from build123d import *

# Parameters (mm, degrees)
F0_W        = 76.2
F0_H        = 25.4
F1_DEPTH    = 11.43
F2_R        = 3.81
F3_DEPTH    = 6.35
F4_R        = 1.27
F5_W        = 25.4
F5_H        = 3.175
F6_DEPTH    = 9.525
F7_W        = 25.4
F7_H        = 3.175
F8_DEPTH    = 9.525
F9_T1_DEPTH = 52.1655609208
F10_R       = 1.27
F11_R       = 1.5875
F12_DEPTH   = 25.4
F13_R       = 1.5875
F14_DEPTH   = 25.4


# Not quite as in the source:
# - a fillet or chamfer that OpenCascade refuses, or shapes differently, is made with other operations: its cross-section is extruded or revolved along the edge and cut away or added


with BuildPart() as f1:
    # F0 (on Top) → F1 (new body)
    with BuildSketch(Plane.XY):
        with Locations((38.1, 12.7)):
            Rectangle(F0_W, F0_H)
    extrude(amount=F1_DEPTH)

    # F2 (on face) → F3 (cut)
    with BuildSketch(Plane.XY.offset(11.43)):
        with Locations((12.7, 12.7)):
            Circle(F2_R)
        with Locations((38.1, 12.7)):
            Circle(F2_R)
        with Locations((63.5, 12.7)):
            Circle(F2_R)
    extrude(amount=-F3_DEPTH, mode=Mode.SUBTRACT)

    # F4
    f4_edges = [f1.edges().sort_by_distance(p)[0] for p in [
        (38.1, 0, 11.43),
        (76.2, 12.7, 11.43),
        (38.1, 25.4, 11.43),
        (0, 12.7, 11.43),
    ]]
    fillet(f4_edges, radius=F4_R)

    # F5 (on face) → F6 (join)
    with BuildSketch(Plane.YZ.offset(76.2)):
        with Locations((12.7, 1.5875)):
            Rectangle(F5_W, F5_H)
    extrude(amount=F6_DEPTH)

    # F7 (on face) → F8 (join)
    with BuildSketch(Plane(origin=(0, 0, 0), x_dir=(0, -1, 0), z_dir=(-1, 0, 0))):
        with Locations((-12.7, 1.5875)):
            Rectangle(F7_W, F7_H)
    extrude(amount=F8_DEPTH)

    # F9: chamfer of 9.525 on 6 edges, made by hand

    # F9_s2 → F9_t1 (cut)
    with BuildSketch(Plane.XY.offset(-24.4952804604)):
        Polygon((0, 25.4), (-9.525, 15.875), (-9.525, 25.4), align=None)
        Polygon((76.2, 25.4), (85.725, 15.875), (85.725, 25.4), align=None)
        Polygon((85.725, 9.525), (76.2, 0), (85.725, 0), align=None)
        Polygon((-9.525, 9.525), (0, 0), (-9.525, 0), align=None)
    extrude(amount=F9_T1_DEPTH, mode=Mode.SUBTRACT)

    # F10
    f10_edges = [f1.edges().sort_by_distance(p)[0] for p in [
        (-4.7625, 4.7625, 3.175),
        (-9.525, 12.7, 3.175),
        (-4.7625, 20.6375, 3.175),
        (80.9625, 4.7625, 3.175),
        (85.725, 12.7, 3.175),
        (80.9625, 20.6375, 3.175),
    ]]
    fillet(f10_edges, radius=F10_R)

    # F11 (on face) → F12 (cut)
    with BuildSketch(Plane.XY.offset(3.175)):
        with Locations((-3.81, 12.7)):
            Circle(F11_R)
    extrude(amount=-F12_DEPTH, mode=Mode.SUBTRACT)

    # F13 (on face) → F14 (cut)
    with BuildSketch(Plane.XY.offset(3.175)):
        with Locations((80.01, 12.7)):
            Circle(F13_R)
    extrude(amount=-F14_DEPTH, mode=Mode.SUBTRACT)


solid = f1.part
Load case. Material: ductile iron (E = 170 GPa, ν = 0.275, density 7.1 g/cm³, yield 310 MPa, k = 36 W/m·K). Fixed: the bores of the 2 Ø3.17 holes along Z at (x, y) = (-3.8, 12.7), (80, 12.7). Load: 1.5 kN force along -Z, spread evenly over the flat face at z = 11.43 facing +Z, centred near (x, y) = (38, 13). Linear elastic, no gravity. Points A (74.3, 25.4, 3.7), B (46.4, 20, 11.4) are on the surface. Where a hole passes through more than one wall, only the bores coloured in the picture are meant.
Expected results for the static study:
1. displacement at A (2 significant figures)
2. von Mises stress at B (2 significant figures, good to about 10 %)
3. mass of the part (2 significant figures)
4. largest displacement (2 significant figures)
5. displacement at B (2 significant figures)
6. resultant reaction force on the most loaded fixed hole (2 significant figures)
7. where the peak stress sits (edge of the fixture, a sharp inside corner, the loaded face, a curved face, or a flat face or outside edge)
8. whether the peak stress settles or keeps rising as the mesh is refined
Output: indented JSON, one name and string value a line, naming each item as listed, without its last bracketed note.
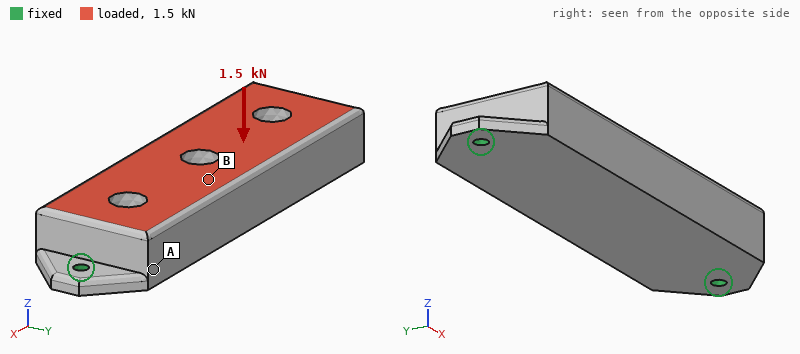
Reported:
{
  "displacement at A": "4.8 µm",
  "von Mises stress at B": "24 MPa",
  "mass of the part": "160 g",
  "largest displacement": "18 µm",
  "displacement at B": "16 µm",
  "resultant reaction force on the most loaded fixed hole": "1.3 kN",
  "where the peak stress sits": "edge of the fixture",
  "whether the peak stress settles or keeps rising as the mesh is refined": "keeps rising"
}
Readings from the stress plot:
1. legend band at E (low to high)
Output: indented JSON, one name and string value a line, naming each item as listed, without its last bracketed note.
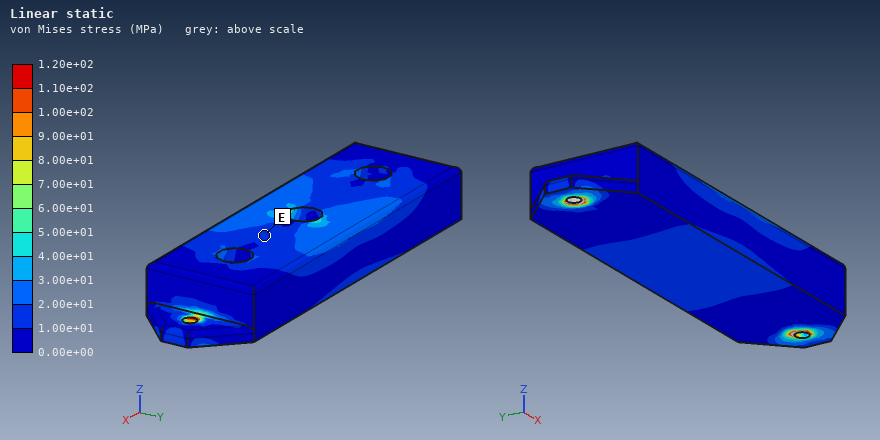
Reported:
{
  "legend band at E": "1.00e+01 to 2.00e+01 MPa"
}
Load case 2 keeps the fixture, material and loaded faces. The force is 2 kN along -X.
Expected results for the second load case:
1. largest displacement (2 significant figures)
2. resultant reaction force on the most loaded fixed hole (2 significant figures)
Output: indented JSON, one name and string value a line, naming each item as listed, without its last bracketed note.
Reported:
{
  "largest displacement": "2.1 µm",
  "resultant reaction force on the most loaded fixed hole": "1.0 kN"
}
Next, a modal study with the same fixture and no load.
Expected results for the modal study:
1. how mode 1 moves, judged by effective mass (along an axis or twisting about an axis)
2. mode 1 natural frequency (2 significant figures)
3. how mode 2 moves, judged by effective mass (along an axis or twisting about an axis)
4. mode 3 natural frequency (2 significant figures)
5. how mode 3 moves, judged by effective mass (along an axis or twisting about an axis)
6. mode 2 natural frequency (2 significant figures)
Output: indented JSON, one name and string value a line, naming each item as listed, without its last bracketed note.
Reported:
{
  "how mode 1 moves, judged by effective mass": "along Y",
  "mode 1 natural frequency": "3200 Hz",
  "how mode 2 moves, judged by effective mass": "along Z",
  "mode 3 natural frequency": "7600 Hz",
  "how mode 3 moves, judged by effective mass": "along Y",
  "mode 2 natural frequency": "4300 Hz"
}
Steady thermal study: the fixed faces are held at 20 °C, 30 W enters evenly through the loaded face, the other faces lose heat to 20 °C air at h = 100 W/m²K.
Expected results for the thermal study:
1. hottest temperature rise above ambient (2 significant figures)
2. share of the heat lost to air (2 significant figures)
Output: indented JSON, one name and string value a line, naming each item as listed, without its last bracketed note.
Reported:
{
  "hottest temperature rise above ambient": "41 K",
  "share of the heat lost to air": "55 %"
}
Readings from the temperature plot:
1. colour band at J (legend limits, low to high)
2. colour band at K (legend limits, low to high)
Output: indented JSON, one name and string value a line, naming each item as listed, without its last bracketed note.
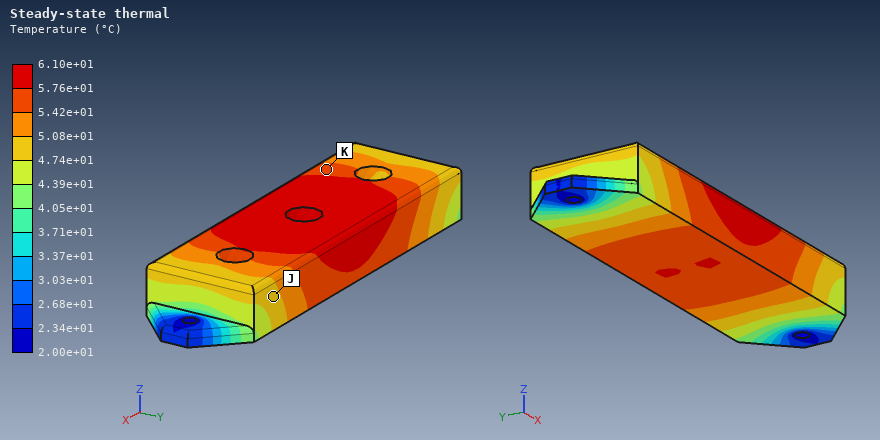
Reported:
{
  "colour band at J": "4.74e+01 to 5.08e+01 °C",
  "colour band at K": "5.42e+01 to 5.76e+01 °C"
}
